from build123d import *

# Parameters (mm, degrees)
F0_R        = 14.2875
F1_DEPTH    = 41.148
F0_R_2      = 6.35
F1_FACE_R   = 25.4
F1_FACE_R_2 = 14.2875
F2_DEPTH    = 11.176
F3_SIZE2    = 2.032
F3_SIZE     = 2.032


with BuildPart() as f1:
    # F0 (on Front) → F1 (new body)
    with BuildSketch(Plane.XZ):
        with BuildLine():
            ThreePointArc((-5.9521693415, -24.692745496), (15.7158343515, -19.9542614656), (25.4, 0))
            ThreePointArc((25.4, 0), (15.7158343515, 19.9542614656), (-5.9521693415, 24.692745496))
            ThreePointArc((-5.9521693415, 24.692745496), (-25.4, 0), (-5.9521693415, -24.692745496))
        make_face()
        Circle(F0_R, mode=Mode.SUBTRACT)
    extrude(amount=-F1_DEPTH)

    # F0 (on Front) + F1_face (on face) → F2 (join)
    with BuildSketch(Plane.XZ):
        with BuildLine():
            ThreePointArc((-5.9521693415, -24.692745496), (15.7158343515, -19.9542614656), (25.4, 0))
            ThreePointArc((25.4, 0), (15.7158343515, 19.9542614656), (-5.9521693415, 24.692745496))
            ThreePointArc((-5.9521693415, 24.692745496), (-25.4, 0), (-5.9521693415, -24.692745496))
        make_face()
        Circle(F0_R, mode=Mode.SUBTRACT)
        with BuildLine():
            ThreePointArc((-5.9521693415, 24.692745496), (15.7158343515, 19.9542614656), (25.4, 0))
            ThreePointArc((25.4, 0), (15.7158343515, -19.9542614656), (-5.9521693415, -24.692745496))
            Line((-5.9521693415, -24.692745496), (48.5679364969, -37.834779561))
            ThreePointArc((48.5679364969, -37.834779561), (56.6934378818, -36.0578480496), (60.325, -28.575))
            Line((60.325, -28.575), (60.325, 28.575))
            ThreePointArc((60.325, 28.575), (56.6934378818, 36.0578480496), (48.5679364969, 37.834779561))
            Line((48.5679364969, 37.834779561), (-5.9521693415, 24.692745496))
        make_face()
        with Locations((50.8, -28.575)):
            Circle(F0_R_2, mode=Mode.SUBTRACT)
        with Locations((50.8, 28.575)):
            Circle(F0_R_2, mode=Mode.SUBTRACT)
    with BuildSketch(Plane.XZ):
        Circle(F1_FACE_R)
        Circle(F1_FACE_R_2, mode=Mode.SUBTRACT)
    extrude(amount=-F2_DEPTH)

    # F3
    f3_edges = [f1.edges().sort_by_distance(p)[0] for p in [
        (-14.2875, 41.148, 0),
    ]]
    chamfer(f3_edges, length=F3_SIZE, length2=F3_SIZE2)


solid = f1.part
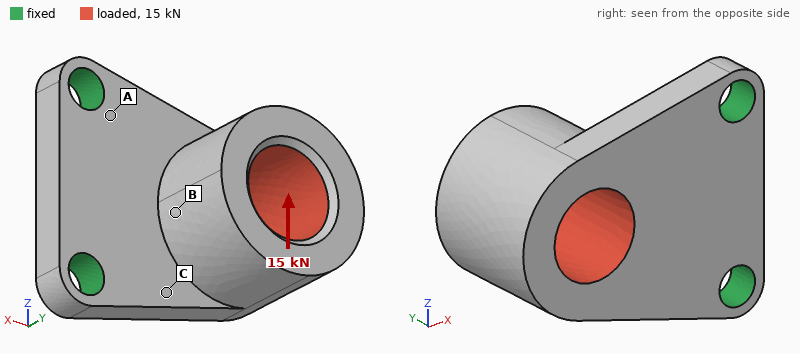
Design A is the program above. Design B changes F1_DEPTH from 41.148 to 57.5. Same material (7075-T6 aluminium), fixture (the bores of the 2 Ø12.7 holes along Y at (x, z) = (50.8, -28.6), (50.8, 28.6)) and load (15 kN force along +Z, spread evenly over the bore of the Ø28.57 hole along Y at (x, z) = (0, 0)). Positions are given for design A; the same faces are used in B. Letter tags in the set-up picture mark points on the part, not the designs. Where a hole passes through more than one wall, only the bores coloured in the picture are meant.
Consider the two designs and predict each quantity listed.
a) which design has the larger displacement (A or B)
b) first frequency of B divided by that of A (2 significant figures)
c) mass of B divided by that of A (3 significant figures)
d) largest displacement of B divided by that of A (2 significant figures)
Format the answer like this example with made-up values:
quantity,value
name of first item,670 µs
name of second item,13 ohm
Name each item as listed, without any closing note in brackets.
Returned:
quantity,value
which design has the larger displacement,B
first frequency of B divided by that of A,0.76
mass of B divided by that of A,1.26
largest displacement of B divided by that of A,1.8
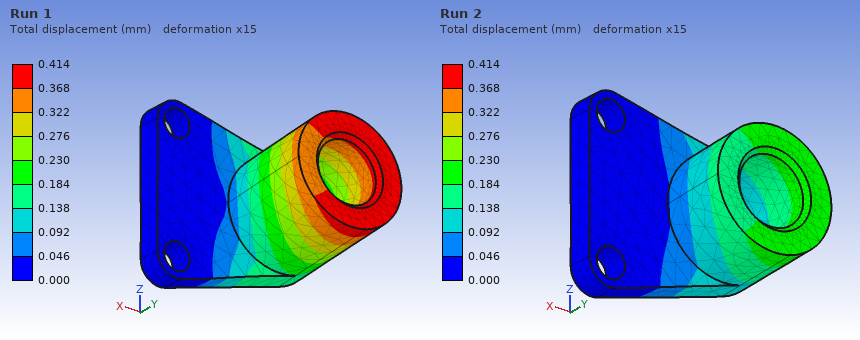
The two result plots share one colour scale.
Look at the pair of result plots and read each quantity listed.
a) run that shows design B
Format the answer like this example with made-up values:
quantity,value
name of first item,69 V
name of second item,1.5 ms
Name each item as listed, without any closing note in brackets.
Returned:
quantity,value
run that shows design B,Run 1
